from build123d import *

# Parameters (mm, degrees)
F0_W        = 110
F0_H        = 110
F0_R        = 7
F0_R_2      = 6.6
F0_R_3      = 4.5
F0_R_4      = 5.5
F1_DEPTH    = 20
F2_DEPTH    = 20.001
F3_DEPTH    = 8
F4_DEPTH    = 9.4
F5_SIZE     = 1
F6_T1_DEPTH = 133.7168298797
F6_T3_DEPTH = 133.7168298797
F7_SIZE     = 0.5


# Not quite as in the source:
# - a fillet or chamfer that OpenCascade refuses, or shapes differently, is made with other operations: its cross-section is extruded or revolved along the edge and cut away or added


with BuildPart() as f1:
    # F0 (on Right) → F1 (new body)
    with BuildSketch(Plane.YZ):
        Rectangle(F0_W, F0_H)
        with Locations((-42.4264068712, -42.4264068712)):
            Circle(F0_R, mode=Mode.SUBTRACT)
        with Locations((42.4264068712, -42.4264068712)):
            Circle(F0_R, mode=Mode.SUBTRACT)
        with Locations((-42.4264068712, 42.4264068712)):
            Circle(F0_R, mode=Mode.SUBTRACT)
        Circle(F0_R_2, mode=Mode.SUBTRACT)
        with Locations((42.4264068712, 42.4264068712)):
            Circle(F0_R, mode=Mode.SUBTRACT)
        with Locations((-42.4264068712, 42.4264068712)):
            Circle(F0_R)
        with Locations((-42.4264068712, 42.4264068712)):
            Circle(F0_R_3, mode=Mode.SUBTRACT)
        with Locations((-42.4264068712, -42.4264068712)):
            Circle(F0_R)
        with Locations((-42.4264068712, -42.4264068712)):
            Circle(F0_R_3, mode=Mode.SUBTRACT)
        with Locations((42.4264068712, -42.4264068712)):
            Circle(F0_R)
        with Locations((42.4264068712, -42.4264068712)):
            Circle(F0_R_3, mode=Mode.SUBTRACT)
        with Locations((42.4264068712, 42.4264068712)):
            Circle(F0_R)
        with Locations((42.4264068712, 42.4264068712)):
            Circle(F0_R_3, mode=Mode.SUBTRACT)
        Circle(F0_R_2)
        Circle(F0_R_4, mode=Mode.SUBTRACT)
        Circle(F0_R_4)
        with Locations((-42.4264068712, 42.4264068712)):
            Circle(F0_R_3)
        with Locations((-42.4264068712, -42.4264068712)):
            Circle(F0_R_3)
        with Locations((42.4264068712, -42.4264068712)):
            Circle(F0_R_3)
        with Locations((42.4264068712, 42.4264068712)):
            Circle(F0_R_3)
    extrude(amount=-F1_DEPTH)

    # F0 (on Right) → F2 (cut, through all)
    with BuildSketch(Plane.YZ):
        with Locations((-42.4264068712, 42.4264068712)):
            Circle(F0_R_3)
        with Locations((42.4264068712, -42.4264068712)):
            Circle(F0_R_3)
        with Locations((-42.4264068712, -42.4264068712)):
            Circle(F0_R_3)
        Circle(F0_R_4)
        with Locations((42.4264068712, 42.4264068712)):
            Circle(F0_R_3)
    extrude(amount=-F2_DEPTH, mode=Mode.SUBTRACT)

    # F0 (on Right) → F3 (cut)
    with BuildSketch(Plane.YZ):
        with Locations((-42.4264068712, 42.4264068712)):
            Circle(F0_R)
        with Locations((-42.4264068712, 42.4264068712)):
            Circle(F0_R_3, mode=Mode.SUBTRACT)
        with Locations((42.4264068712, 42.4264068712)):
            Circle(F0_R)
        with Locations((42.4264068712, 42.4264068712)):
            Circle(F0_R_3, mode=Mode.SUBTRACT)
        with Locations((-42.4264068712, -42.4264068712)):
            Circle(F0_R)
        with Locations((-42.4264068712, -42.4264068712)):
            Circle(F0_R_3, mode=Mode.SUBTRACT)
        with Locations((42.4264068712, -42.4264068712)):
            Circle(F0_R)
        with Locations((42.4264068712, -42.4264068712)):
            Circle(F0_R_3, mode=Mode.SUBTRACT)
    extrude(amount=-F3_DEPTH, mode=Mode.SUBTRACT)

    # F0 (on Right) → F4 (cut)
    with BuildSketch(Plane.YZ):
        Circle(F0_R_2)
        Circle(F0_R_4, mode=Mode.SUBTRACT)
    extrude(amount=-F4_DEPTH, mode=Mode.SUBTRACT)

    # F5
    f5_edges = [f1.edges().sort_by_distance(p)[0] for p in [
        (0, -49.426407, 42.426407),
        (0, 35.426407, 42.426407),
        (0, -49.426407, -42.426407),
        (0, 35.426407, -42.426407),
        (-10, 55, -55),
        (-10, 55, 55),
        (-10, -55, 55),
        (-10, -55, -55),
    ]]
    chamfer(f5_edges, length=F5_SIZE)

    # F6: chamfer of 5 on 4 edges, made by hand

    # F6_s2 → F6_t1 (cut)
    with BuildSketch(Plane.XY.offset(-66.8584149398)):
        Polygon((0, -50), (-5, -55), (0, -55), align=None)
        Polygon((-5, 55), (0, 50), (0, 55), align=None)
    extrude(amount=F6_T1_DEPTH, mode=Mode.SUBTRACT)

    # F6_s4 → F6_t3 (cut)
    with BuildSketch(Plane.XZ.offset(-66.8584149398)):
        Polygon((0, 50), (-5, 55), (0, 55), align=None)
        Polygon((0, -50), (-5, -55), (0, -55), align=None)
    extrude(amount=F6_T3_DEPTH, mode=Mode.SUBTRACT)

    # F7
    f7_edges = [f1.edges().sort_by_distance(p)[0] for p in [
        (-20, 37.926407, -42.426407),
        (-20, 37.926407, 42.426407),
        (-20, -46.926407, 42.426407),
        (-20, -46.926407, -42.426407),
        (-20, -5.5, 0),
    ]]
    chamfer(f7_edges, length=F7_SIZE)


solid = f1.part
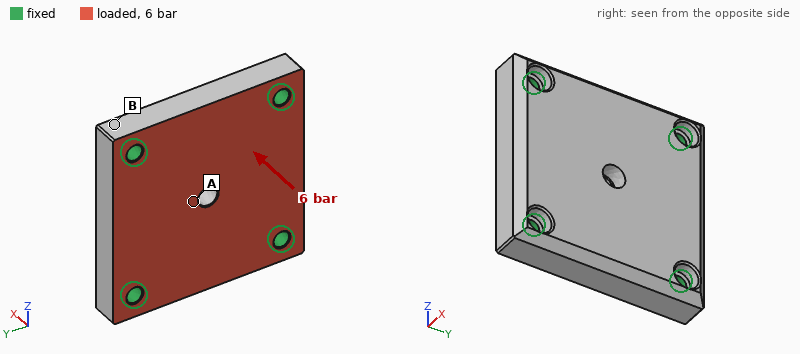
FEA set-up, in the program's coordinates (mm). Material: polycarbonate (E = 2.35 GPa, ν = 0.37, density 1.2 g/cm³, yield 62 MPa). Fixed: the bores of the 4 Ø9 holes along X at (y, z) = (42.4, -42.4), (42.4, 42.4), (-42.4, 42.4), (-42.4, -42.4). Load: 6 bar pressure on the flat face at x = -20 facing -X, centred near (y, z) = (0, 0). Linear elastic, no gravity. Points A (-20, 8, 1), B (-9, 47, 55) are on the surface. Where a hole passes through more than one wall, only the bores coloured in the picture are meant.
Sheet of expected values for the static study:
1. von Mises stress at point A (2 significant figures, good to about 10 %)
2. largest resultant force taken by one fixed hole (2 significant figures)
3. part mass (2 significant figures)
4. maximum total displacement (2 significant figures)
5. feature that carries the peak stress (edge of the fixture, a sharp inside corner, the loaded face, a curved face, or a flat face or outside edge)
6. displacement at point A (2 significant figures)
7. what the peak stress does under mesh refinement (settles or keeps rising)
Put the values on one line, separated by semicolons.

4.7 MPa; 1.8 kN; 270 g; 0.27 mm; edge of the fixture; 0.26 mm; keeps rising
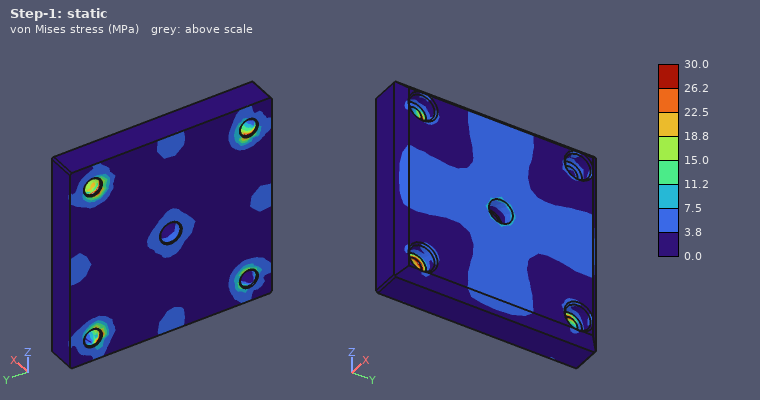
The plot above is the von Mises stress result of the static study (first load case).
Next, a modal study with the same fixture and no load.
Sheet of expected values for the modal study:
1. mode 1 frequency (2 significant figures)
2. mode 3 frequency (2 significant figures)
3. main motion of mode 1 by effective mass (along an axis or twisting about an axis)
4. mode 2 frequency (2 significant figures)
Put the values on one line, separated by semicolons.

1900 Hz; 2800 Hz; along X; 2800 Hz
